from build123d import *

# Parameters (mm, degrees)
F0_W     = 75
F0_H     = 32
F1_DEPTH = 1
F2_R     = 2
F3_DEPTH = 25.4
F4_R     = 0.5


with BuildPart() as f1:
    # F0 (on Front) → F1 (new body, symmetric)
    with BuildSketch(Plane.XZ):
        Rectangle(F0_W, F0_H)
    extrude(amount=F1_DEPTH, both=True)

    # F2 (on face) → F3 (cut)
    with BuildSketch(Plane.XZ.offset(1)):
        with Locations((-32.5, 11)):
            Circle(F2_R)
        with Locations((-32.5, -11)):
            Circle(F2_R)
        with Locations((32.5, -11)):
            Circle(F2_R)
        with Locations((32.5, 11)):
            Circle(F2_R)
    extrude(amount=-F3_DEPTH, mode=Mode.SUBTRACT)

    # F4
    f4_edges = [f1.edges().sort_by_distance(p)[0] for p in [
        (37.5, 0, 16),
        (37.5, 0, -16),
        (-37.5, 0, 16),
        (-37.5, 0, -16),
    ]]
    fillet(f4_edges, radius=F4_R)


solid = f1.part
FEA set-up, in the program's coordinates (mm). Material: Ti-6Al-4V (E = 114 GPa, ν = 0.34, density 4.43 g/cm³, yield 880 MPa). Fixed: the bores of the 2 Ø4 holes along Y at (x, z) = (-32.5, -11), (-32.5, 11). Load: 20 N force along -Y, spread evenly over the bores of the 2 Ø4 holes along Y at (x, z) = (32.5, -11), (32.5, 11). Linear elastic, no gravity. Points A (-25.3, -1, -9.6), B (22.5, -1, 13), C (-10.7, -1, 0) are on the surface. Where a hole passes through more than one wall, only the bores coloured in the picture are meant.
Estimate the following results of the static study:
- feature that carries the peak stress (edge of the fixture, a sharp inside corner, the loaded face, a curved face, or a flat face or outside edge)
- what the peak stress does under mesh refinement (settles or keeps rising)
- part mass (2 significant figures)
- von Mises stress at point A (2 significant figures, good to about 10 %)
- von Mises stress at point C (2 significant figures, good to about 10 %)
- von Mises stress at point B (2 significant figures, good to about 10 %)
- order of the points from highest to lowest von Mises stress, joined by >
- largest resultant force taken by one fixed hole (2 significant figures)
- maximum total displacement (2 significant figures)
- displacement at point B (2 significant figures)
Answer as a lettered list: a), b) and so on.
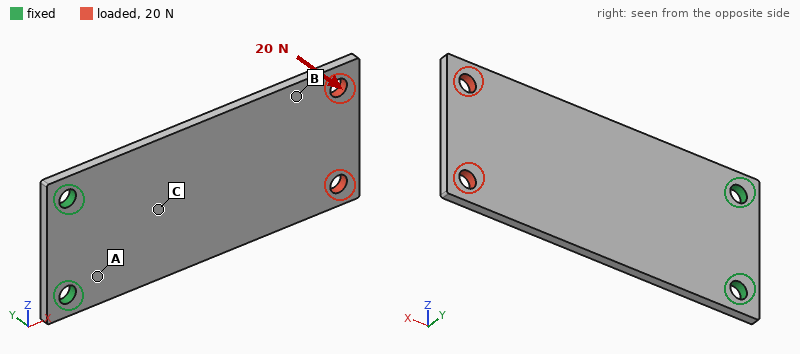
a) edge of the fixture
b) keeps rising
c) 21 g
d) 51 MPa
e) 39 MPa
f) 10 MPa
g) A > C > B
h) 10 N
i) 0.80 mm
j) 0.55 mm
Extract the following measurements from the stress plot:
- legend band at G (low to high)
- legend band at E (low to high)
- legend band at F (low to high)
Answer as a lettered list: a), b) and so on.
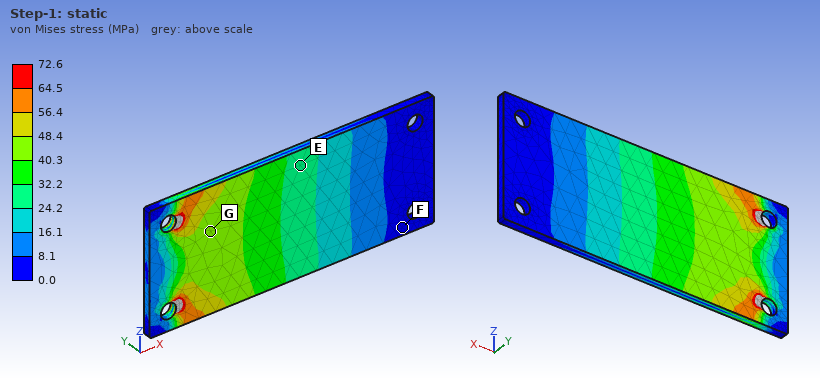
a) 40.3 to 48.4 MPa
b) 24.2 to 32.2 MPa
c) 0.0 to 8.1 MPa
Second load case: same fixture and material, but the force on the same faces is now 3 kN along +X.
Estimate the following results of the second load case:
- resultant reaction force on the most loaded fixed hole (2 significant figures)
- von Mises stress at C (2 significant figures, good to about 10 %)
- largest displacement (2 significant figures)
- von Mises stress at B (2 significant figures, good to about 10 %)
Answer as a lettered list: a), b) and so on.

a) 1.5 kN
b) 45 MPa
c) 34 µm
d) 58 MPa
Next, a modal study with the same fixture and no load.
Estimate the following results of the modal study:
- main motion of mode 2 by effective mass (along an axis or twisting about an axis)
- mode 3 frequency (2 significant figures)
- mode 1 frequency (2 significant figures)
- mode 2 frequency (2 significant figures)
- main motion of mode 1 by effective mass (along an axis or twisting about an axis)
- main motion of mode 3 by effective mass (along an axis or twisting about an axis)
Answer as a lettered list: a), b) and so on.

a) twisting about X
b) 2200 Hz
c) 350 Hz
d) 1600 Hz
e) along Y
f) along Y
